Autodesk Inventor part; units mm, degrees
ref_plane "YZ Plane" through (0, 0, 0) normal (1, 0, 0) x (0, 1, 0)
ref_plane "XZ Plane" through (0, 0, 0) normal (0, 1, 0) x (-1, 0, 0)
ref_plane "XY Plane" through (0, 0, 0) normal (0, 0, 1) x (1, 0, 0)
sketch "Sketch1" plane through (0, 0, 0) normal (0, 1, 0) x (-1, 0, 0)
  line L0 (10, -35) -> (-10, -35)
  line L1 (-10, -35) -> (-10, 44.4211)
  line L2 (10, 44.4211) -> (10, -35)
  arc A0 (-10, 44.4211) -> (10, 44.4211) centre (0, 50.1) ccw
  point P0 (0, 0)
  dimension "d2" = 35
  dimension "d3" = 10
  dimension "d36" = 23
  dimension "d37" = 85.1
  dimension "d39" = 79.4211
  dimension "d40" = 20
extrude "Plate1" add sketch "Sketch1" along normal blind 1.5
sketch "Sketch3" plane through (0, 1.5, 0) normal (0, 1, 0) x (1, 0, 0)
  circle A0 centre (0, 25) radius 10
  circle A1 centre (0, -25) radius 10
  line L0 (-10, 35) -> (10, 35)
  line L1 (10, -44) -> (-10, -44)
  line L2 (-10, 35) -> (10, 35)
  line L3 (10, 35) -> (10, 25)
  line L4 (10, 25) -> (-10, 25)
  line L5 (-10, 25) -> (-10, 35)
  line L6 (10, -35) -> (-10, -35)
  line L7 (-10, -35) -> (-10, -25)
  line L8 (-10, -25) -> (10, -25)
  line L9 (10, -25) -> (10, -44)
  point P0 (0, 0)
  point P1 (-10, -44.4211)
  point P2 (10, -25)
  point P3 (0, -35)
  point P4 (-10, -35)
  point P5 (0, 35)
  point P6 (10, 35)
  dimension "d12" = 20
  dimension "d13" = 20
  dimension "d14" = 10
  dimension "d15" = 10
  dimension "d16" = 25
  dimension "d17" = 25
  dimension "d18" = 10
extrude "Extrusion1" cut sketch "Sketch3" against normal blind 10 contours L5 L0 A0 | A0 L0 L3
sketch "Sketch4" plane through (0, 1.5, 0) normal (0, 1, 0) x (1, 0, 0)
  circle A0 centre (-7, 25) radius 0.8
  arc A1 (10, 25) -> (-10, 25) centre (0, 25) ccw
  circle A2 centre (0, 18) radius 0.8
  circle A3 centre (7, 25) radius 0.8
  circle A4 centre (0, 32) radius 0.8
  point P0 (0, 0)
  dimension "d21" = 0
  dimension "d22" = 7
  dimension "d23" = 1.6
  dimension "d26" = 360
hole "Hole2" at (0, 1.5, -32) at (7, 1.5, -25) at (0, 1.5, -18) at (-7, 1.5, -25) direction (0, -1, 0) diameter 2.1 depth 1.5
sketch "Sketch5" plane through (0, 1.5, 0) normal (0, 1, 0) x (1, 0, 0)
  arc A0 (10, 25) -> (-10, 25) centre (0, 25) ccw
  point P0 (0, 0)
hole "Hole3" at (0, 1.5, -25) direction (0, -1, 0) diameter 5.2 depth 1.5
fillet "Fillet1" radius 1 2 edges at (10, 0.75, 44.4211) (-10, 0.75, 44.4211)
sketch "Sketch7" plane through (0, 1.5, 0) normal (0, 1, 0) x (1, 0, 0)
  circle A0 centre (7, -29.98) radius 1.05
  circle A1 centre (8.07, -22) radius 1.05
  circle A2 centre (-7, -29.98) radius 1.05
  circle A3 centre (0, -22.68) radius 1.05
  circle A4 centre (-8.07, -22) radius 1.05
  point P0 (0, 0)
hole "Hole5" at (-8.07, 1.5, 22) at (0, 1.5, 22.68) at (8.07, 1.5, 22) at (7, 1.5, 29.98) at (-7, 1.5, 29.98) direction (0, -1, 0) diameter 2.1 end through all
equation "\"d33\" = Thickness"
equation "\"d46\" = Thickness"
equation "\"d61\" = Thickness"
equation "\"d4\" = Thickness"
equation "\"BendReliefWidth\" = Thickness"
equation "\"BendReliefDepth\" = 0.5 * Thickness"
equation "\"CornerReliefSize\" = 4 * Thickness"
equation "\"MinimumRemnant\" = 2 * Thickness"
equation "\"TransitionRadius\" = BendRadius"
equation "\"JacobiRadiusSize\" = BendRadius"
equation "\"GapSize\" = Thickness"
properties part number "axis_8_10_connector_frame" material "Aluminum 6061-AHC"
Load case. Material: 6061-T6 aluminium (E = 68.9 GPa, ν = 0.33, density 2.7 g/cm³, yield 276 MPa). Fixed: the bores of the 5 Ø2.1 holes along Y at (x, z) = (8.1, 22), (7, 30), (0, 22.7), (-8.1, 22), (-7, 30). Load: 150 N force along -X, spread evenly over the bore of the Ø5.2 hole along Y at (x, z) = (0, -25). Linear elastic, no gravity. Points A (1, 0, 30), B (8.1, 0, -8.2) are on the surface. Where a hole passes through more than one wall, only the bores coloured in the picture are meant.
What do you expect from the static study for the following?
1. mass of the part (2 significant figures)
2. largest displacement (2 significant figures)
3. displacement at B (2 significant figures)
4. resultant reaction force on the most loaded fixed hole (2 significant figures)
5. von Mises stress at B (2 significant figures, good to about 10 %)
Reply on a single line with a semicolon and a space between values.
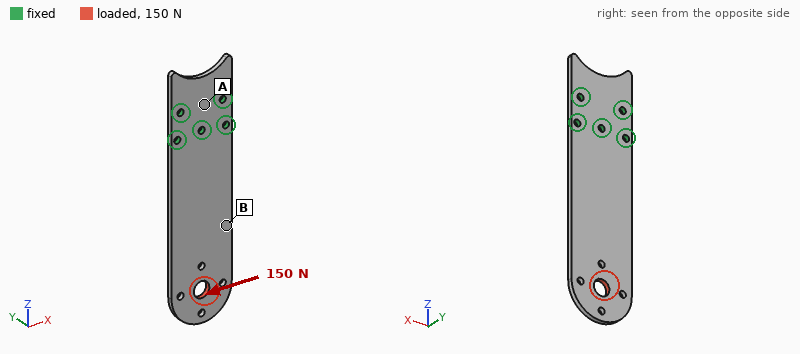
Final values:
5.7 g; 0.11 mm; 0.046 mm; 410 N; 21 MPa
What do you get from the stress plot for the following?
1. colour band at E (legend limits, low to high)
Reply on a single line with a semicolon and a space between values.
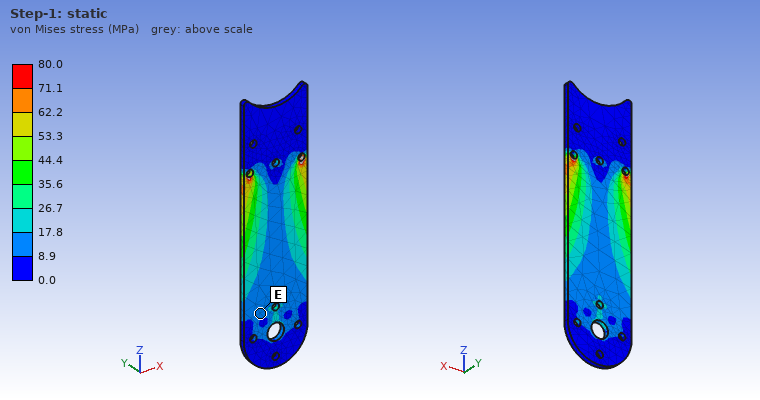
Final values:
8.9 to 17.8 MPa
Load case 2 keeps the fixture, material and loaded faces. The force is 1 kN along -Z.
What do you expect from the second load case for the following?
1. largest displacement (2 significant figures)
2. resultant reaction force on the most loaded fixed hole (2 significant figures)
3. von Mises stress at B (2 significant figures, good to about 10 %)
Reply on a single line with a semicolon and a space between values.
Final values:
29 µm; 320 N; 34 MPa
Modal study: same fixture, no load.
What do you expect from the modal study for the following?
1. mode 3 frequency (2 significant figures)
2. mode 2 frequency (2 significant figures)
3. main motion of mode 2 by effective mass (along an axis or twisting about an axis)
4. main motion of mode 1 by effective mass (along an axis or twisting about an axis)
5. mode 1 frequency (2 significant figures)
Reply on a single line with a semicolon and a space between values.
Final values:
2600 Hz; 2400 Hz; twisting about Z; along Y; 430 Hz
